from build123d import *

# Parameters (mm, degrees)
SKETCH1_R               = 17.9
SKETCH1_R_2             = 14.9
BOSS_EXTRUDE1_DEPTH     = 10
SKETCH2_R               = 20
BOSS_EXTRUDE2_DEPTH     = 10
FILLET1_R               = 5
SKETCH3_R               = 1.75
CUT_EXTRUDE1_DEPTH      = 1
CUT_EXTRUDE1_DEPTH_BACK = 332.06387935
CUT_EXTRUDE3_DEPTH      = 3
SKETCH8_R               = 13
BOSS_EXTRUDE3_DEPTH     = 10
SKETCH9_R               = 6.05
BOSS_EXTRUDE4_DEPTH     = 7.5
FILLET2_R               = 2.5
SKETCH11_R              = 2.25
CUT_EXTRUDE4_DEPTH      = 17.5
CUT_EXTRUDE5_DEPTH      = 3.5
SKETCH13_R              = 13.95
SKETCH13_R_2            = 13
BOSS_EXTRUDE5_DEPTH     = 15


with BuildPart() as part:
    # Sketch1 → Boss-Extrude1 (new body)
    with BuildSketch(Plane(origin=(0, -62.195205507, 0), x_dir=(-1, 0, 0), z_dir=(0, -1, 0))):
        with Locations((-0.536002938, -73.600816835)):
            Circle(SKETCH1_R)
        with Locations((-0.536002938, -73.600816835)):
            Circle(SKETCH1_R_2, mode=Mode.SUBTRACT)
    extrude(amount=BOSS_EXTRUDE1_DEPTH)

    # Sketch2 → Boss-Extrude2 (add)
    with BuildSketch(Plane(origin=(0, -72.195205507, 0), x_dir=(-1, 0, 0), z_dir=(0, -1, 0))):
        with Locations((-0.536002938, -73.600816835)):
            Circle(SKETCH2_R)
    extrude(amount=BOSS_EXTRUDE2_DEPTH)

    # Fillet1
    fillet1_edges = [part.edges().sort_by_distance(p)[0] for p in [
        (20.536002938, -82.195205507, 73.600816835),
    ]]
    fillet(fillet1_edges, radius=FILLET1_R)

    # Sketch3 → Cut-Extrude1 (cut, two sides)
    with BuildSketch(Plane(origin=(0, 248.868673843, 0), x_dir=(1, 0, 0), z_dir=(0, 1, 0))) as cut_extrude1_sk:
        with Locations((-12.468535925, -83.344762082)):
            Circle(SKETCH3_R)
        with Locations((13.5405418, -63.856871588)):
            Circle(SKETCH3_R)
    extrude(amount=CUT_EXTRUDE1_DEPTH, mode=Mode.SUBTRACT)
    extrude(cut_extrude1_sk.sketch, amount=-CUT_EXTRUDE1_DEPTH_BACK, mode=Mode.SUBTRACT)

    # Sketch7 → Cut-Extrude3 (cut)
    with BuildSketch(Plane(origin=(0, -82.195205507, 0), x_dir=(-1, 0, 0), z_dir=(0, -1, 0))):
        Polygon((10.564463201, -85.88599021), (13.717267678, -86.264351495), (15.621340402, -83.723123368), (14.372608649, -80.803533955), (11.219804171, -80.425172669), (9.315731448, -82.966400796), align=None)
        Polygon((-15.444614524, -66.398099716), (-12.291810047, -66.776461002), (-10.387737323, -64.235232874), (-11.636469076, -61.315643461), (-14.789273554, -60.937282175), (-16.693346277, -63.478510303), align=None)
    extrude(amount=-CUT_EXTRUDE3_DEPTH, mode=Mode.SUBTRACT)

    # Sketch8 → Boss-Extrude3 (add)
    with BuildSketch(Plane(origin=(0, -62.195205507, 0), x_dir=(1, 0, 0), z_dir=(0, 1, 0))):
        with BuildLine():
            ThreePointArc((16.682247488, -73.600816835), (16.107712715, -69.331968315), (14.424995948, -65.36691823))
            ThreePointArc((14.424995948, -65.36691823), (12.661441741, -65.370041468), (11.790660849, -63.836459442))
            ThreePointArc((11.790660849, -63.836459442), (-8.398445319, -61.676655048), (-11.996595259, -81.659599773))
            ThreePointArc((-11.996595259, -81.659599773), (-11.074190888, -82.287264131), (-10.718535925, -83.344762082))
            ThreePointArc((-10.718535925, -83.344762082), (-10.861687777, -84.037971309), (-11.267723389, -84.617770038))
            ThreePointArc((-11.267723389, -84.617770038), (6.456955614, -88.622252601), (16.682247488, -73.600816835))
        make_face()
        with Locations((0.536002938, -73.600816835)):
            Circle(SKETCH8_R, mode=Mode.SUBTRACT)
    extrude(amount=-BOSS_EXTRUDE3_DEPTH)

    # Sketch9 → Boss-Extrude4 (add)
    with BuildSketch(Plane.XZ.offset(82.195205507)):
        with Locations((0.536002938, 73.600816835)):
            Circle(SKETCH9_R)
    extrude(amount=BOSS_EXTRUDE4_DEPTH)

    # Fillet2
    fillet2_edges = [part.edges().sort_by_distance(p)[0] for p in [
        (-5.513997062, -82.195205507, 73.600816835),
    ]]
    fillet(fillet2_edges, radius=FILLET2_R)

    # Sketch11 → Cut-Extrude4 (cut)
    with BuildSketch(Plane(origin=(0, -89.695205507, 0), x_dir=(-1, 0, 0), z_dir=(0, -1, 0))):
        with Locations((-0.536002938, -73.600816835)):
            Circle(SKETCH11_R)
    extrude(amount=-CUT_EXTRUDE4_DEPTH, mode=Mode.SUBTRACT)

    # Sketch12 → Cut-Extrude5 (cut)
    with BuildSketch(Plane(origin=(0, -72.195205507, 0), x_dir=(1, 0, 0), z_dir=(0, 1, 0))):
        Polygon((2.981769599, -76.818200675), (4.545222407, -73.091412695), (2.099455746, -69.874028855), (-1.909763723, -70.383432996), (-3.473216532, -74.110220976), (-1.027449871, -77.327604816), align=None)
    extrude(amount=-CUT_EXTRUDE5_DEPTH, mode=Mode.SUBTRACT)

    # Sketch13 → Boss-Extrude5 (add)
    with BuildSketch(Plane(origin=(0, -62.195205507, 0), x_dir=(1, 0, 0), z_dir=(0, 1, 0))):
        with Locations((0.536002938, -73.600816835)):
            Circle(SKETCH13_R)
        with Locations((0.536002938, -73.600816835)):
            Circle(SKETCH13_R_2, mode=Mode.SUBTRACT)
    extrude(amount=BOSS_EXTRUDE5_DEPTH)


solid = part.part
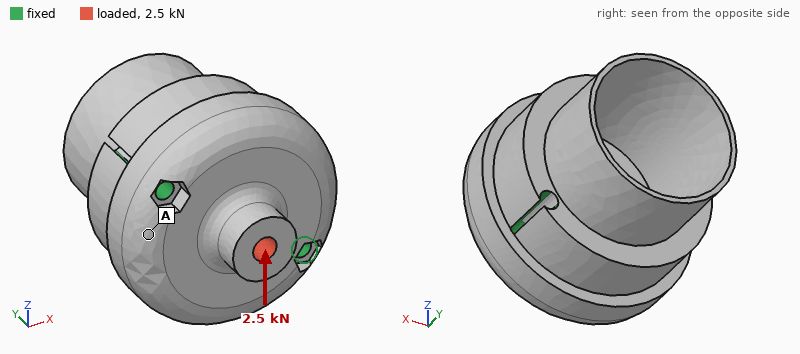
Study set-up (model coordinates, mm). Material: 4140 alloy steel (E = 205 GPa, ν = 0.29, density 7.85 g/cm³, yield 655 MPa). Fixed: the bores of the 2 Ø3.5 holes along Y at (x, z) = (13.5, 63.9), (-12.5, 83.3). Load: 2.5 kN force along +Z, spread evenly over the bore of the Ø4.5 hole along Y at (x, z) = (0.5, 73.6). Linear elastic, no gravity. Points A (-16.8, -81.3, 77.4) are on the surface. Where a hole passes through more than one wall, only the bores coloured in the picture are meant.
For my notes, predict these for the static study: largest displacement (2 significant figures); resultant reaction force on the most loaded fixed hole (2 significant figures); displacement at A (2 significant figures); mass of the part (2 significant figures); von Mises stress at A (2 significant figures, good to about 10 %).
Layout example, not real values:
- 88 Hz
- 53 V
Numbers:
- 4.0 µm
- 1.3 kN
- 0.85 µm
- 140 g
- 6.5 MPa
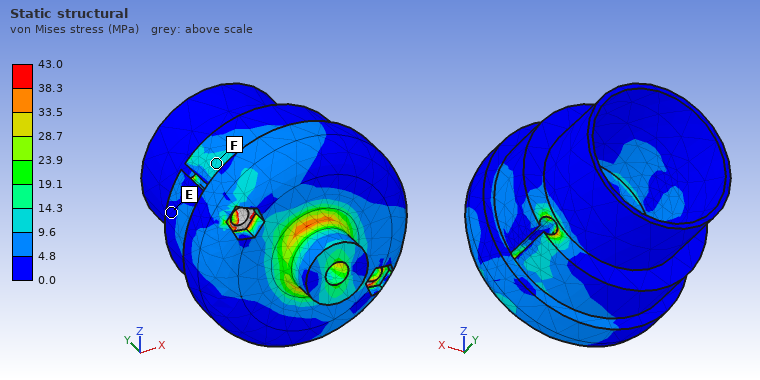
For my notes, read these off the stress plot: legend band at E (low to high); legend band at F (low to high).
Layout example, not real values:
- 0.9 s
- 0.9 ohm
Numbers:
- 0.0 to 4.8 MPa
- 9.6 to 14.3 MPa
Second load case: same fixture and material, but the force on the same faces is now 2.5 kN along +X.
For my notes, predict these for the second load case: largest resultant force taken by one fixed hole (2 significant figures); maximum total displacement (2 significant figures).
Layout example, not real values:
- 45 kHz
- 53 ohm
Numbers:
- 1.3 kN
- 3.5 µm
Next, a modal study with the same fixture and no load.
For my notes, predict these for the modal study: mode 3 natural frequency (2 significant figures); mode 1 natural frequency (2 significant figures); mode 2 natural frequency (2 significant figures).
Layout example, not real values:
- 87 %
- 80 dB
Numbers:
- 17 kHz
- 16 kHz
- 16 kHz
